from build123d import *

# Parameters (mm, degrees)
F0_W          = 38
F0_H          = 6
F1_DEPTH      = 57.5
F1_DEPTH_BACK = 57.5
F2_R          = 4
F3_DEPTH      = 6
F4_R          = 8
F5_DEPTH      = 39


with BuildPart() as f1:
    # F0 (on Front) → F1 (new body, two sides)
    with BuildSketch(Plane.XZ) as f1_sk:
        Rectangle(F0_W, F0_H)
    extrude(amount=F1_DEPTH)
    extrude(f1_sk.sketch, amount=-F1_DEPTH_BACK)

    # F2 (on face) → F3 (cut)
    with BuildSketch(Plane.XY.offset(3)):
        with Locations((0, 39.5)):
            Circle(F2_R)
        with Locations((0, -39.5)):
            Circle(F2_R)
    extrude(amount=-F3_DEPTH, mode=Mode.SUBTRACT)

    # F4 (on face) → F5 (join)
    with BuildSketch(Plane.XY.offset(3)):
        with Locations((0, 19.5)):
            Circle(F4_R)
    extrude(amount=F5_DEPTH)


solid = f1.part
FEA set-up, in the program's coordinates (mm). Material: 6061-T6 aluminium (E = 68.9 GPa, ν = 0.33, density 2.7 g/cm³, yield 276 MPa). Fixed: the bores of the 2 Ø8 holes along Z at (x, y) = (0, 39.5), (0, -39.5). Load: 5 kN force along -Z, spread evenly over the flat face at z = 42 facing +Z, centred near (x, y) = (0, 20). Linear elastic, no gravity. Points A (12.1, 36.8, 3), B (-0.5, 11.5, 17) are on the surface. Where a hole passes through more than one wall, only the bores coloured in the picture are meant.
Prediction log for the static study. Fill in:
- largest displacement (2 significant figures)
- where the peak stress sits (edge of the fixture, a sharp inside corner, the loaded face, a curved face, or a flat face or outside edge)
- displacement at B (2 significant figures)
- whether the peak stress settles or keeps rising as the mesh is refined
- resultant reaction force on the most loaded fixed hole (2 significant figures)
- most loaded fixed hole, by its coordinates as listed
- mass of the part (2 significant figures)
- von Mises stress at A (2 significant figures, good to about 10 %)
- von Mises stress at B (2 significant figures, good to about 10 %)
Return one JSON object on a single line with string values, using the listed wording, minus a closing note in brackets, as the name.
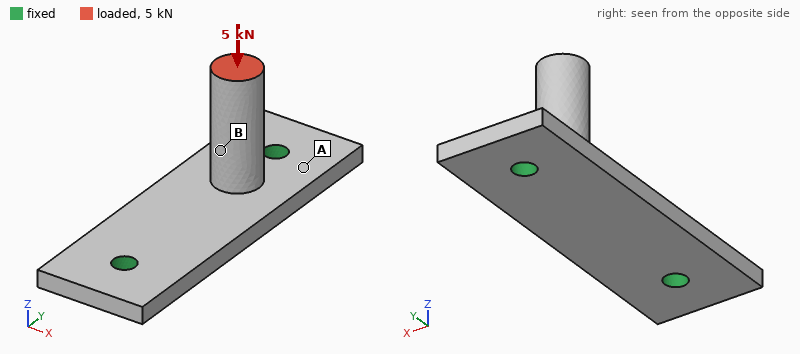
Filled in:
{"largest displacement": "0.27 mm", "where the peak stress sits": "edge of the fixture", "displacement at B": "0.18 mm", "whether the peak stress settles or keeps rising as the mesh is refined": "keeps rising", "resultant reaction force on the most loaded fixed hole": "4.1 kN", "most loaded fixed hole, by its coordinates as listed": "(0, 39.5)", "mass of the part": "90 g", "von Mises stress at A": "67 MPa", "von Mises stress at B": "24 MPa"}
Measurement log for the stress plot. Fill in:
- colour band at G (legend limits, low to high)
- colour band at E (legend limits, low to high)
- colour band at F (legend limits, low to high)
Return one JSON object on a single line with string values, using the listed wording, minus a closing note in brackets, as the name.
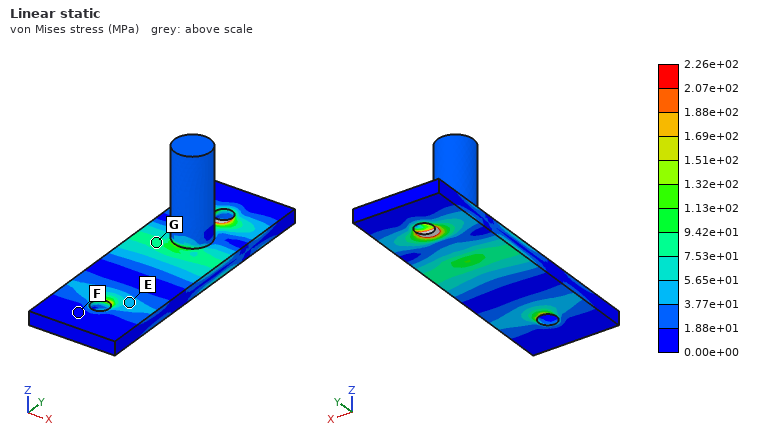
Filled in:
{"colour band at G": "7.53e+01 to 9.42e+01 MPa", "colour band at E": "3.77e+01 to 5.65e+01 MPa", "colour band at F": "0.00e+00 to 1.88e+01 MPa"}
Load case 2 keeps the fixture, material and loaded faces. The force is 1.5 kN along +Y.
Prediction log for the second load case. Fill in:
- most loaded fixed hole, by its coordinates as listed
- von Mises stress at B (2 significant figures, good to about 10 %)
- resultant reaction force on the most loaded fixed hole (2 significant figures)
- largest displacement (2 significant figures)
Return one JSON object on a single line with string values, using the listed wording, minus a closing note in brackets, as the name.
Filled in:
{"most loaded fixed hole, by its coordinates as listed": "(0, 39.5)", "von Mises stress at B": "93 MPa", "resultant reaction force on the most loaded fixed hole": "1.4 kN", "largest displacement": "0.47 mm"}
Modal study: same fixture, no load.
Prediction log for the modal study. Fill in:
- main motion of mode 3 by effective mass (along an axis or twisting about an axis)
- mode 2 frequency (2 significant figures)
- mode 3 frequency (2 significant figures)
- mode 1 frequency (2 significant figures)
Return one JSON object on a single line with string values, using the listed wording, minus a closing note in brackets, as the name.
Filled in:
{"main motion of mode 3 by effective mass": "along Z", "mode 2 frequency": "3000 Hz", "mode 3 frequency": "6700 Hz", "mode 1 frequency": "2900 Hz"}
